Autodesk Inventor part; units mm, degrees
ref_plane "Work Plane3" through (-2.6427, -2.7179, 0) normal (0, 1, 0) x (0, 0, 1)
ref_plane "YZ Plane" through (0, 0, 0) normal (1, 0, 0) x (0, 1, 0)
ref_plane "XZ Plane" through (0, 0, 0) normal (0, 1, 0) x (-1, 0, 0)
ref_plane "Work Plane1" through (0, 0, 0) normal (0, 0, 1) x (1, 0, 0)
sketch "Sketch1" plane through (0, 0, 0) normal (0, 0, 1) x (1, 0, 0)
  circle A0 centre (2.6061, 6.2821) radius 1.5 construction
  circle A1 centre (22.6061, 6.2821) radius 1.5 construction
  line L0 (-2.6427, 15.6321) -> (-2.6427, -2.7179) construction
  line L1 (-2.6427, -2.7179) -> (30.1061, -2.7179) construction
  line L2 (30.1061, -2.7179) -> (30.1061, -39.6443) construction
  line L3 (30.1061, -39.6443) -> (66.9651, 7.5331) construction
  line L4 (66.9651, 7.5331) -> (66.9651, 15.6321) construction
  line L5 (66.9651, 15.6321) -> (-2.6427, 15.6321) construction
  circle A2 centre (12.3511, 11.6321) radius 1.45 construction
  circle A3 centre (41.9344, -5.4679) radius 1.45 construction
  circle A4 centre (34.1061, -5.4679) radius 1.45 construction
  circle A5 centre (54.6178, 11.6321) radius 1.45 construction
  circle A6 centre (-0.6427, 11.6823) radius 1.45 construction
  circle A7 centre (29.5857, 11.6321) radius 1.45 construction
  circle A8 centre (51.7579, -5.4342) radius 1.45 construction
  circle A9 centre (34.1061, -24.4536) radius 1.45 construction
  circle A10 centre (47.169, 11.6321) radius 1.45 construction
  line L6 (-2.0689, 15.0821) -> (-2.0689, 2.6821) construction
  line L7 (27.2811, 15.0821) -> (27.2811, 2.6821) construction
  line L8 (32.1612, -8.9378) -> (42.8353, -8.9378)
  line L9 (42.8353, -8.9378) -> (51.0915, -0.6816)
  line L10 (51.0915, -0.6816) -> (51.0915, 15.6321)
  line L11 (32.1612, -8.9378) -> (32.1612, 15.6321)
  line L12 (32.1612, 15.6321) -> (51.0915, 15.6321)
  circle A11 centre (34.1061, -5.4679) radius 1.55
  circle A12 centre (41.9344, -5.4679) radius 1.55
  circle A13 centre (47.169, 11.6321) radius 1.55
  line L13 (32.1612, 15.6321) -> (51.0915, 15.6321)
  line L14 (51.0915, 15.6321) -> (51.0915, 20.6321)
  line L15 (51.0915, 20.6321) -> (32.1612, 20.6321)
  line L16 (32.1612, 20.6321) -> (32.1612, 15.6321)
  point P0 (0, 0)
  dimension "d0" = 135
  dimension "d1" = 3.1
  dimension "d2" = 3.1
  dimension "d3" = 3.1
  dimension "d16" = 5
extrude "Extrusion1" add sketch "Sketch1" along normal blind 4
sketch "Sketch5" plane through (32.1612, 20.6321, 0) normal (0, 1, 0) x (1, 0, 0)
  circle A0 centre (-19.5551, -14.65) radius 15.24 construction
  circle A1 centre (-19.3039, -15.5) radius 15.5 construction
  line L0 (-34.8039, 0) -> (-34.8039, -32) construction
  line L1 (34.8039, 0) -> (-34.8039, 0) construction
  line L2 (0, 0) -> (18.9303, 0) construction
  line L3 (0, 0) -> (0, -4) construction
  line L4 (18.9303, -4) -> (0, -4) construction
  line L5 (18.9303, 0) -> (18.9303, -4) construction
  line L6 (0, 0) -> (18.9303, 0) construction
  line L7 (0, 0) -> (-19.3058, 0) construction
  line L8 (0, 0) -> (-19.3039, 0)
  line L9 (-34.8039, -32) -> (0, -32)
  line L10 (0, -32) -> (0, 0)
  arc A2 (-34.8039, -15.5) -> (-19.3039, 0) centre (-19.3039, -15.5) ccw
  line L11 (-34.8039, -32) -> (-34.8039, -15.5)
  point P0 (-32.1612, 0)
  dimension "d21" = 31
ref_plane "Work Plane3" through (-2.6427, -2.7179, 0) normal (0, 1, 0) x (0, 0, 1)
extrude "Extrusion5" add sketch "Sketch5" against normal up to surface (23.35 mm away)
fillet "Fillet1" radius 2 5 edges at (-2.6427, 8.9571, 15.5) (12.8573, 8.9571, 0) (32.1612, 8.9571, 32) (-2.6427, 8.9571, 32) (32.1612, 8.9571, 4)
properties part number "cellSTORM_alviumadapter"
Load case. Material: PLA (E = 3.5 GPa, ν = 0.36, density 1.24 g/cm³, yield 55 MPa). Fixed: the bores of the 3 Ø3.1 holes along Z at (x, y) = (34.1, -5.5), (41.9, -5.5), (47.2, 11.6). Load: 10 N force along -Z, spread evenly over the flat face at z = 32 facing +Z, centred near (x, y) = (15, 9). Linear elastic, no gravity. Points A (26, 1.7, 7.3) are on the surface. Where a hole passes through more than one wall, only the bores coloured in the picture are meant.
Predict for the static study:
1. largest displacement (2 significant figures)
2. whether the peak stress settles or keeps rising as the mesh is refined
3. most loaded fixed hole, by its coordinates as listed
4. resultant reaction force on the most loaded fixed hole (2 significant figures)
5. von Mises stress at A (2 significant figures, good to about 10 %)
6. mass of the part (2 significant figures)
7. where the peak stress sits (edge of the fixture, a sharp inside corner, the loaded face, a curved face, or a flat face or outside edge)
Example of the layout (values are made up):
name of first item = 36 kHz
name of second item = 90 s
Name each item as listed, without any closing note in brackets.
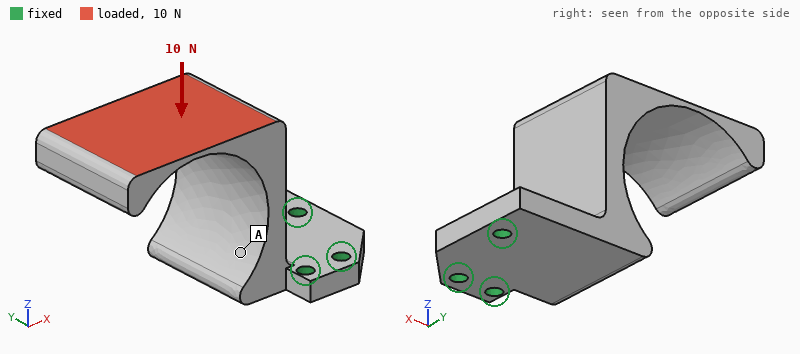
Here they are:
largest displacement = 0.82 mm
whether the peak stress settles or keeps rising as the mesh is refined = keeps rising
most loaded fixed hole, by its coordinates as listed = (34.1, -5.5)
resultant reaction force on the most loaded fixed hole = 17 N
von Mises stress at A = 1.0 MPa
mass of the part = 11 g
where the peak stress sits = edge of the fixture
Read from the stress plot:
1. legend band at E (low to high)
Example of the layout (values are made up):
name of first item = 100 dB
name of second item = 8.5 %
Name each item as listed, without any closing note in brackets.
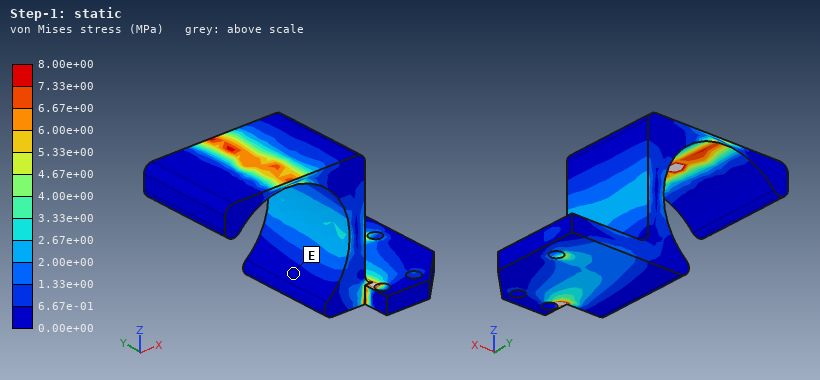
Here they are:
legend band at E = 0.00e+00 to 6.67e-01 MPa
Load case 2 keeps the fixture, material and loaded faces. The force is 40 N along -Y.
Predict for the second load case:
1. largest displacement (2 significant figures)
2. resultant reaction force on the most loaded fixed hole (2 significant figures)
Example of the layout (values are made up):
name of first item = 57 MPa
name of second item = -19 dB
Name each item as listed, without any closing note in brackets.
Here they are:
largest displacement = 0.69 mm
resultant reaction force on the most loaded fixed hole = 69 N
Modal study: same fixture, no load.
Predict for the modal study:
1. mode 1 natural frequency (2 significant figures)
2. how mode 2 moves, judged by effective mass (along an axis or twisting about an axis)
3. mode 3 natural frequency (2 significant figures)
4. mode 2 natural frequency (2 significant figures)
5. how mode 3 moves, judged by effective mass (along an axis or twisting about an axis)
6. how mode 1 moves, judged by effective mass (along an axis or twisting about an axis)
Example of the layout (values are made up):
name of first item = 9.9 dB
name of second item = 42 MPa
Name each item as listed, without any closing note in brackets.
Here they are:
mode 1 natural frequency = 290 Hz
how mode 2 moves, judged by effective mass = along X
mode 3 natural frequency = 770 Hz
mode 2 natural frequency = 520 Hz
how mode 3 moves, judged by effective mass = along Y
how mode 1 moves, judged by effective mass = along Z
